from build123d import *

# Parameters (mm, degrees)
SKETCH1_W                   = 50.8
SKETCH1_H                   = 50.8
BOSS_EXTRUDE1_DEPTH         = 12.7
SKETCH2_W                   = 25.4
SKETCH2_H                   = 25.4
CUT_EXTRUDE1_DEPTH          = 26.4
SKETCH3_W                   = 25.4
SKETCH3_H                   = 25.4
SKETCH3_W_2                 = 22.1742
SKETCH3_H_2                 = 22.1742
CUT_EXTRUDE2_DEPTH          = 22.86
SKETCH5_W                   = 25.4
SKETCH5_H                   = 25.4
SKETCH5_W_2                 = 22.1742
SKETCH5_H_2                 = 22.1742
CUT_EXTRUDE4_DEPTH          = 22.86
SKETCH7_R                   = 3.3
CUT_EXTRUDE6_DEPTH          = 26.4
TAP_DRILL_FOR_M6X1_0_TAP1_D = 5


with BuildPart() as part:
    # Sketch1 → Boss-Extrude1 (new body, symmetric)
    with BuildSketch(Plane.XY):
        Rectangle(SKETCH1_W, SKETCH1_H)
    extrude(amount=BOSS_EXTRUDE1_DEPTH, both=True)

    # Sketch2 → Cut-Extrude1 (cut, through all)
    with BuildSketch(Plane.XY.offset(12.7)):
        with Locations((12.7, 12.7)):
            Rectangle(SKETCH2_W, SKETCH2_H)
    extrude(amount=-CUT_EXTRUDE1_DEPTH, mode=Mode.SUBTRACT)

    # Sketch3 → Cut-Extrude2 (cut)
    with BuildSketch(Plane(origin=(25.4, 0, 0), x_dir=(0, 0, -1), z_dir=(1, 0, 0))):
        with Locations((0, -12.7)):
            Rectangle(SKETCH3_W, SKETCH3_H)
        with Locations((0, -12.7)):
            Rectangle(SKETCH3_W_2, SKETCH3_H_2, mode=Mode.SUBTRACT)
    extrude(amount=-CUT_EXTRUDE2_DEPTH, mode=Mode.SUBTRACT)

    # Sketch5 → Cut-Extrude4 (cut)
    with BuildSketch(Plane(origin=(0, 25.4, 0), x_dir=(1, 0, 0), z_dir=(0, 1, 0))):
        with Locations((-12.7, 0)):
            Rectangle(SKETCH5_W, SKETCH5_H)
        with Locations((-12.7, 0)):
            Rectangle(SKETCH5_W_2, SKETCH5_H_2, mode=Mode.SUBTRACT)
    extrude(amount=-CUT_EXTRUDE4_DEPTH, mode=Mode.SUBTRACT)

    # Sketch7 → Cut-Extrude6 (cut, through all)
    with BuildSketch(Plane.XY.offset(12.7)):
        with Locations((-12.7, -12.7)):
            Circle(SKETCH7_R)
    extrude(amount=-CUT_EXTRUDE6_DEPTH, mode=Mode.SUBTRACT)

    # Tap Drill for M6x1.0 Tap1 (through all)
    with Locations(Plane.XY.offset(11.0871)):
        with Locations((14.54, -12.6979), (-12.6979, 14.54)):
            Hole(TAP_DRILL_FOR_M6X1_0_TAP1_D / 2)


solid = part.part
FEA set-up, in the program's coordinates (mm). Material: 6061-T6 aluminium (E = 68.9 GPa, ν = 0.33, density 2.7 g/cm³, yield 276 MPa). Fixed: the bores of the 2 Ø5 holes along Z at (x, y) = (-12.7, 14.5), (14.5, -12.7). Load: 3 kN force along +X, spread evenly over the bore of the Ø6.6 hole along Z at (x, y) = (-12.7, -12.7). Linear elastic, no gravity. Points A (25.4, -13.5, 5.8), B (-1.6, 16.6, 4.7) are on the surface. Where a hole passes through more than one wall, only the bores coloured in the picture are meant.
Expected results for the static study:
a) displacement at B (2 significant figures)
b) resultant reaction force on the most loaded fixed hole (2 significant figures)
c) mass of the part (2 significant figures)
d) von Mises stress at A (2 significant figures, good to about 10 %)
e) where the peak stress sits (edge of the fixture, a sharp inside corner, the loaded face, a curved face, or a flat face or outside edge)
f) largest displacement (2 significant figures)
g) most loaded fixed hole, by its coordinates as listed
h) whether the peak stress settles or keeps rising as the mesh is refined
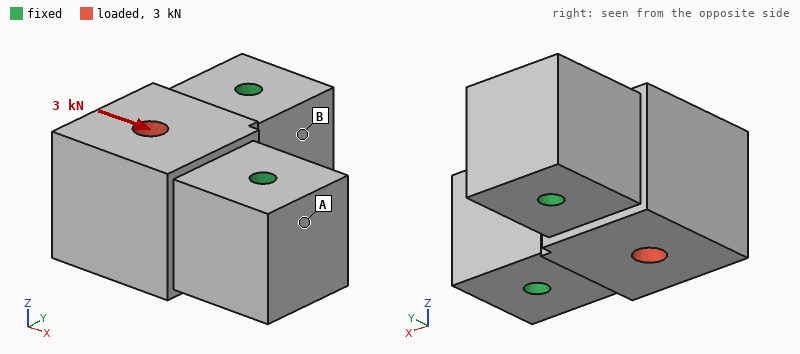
0.64 µm
2.7 kN
110 g
3.1 MPa
edge of the fixture
3.2 µm
(14.5, -12.7)
keeps rising
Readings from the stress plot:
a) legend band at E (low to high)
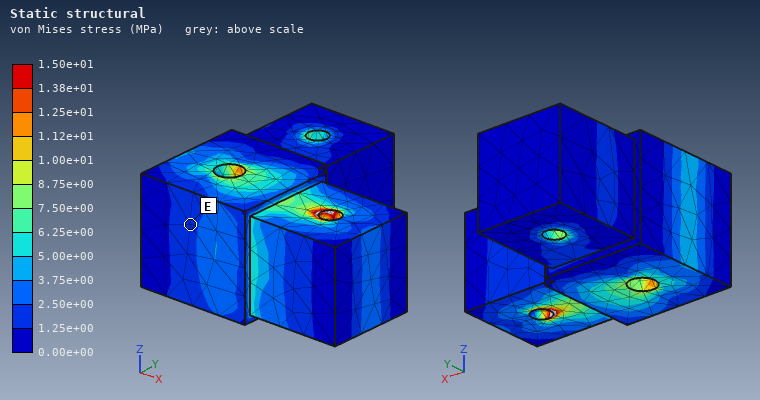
1.25e+00 to 2.50e+00 MPa
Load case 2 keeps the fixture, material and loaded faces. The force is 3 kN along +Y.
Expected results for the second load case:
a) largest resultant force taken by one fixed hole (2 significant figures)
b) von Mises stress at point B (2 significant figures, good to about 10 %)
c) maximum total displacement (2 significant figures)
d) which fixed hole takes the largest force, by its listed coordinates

2.7 kN
2.0 MPa
3.2 µm
(-12.7, 14.5)
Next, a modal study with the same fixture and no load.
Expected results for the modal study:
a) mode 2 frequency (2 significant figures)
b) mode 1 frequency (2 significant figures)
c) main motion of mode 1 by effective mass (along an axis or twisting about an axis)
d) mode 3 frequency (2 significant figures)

24 kHz
12 kHz
along Z
28 kHz
